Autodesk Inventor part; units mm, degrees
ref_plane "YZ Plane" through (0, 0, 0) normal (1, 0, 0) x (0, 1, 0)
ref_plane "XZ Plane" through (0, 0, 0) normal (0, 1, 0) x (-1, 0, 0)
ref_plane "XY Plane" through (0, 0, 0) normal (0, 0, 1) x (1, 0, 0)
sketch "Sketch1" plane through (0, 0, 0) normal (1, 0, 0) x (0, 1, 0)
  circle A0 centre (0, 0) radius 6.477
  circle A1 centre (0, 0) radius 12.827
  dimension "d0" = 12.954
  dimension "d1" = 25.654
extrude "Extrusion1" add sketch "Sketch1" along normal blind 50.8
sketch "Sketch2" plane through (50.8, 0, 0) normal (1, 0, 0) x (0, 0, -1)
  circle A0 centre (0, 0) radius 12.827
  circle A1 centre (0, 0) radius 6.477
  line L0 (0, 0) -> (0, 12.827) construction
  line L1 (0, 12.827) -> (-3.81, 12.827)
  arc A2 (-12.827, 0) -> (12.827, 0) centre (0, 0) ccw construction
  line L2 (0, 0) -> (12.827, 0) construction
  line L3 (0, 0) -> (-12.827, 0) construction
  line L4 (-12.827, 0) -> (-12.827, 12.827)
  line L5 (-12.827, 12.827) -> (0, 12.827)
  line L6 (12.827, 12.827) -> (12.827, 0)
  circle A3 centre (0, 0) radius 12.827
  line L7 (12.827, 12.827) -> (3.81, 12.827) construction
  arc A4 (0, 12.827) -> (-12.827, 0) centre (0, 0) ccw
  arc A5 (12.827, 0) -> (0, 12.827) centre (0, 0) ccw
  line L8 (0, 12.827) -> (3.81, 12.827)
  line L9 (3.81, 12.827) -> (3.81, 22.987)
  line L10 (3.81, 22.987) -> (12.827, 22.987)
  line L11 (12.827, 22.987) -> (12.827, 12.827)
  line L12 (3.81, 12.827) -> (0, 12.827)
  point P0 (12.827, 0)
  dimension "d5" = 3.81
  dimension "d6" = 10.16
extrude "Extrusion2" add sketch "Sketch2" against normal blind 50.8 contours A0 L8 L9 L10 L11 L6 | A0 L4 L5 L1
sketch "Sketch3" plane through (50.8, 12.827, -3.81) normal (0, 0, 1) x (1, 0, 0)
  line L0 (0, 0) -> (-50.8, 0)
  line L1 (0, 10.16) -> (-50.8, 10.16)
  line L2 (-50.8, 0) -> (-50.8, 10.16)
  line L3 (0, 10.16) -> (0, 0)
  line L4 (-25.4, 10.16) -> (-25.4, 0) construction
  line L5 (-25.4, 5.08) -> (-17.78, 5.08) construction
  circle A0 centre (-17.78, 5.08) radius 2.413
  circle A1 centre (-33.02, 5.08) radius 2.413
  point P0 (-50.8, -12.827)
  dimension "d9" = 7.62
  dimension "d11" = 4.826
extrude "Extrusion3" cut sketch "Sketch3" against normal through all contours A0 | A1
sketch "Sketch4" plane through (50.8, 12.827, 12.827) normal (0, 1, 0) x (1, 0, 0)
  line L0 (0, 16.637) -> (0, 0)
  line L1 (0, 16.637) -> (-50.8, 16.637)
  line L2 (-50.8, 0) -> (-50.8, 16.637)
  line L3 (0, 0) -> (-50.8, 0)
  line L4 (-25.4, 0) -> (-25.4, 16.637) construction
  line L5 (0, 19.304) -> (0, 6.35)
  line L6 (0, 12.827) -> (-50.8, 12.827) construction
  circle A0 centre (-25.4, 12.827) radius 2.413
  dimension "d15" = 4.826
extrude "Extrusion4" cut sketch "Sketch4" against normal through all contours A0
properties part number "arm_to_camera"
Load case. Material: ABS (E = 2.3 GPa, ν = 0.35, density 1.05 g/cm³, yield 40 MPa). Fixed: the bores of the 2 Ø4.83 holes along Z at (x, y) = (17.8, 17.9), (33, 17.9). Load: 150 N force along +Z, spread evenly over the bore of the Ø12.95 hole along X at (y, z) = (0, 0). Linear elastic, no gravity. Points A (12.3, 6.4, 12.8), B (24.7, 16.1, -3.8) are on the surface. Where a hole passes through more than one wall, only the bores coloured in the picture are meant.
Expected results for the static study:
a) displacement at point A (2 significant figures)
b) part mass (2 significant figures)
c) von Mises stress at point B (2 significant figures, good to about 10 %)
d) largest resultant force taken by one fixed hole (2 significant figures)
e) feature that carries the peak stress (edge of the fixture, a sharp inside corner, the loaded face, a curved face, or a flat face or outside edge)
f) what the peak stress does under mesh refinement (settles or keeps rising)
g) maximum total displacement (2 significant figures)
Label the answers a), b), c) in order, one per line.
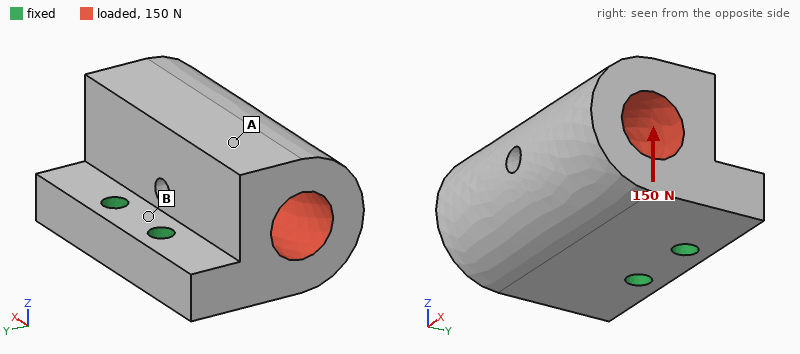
a) 0.093 mm
b) 29 g
c) 2.2 MPa
d) 75 N
e) edge of the fixture
f) keeps rising
g) 0.12 mm
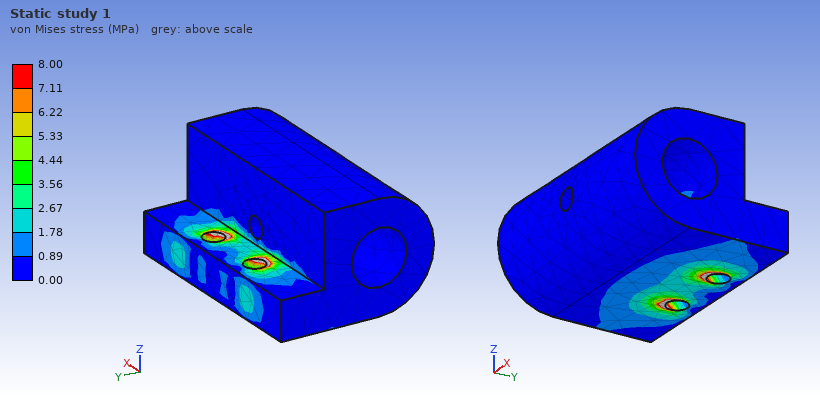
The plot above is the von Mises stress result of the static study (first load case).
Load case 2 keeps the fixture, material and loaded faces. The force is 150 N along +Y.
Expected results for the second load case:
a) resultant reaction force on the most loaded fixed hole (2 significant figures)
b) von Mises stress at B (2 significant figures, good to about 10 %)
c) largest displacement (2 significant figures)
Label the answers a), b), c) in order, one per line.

a) 75 N
b) 1.3 MPa
c) 72 µm
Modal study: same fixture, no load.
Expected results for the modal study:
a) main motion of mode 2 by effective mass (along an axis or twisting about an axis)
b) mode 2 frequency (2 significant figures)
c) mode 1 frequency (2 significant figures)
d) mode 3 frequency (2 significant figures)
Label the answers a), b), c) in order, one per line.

a) along X
b) 2100 Hz
c) 1200 Hz
d) 2600 Hz
